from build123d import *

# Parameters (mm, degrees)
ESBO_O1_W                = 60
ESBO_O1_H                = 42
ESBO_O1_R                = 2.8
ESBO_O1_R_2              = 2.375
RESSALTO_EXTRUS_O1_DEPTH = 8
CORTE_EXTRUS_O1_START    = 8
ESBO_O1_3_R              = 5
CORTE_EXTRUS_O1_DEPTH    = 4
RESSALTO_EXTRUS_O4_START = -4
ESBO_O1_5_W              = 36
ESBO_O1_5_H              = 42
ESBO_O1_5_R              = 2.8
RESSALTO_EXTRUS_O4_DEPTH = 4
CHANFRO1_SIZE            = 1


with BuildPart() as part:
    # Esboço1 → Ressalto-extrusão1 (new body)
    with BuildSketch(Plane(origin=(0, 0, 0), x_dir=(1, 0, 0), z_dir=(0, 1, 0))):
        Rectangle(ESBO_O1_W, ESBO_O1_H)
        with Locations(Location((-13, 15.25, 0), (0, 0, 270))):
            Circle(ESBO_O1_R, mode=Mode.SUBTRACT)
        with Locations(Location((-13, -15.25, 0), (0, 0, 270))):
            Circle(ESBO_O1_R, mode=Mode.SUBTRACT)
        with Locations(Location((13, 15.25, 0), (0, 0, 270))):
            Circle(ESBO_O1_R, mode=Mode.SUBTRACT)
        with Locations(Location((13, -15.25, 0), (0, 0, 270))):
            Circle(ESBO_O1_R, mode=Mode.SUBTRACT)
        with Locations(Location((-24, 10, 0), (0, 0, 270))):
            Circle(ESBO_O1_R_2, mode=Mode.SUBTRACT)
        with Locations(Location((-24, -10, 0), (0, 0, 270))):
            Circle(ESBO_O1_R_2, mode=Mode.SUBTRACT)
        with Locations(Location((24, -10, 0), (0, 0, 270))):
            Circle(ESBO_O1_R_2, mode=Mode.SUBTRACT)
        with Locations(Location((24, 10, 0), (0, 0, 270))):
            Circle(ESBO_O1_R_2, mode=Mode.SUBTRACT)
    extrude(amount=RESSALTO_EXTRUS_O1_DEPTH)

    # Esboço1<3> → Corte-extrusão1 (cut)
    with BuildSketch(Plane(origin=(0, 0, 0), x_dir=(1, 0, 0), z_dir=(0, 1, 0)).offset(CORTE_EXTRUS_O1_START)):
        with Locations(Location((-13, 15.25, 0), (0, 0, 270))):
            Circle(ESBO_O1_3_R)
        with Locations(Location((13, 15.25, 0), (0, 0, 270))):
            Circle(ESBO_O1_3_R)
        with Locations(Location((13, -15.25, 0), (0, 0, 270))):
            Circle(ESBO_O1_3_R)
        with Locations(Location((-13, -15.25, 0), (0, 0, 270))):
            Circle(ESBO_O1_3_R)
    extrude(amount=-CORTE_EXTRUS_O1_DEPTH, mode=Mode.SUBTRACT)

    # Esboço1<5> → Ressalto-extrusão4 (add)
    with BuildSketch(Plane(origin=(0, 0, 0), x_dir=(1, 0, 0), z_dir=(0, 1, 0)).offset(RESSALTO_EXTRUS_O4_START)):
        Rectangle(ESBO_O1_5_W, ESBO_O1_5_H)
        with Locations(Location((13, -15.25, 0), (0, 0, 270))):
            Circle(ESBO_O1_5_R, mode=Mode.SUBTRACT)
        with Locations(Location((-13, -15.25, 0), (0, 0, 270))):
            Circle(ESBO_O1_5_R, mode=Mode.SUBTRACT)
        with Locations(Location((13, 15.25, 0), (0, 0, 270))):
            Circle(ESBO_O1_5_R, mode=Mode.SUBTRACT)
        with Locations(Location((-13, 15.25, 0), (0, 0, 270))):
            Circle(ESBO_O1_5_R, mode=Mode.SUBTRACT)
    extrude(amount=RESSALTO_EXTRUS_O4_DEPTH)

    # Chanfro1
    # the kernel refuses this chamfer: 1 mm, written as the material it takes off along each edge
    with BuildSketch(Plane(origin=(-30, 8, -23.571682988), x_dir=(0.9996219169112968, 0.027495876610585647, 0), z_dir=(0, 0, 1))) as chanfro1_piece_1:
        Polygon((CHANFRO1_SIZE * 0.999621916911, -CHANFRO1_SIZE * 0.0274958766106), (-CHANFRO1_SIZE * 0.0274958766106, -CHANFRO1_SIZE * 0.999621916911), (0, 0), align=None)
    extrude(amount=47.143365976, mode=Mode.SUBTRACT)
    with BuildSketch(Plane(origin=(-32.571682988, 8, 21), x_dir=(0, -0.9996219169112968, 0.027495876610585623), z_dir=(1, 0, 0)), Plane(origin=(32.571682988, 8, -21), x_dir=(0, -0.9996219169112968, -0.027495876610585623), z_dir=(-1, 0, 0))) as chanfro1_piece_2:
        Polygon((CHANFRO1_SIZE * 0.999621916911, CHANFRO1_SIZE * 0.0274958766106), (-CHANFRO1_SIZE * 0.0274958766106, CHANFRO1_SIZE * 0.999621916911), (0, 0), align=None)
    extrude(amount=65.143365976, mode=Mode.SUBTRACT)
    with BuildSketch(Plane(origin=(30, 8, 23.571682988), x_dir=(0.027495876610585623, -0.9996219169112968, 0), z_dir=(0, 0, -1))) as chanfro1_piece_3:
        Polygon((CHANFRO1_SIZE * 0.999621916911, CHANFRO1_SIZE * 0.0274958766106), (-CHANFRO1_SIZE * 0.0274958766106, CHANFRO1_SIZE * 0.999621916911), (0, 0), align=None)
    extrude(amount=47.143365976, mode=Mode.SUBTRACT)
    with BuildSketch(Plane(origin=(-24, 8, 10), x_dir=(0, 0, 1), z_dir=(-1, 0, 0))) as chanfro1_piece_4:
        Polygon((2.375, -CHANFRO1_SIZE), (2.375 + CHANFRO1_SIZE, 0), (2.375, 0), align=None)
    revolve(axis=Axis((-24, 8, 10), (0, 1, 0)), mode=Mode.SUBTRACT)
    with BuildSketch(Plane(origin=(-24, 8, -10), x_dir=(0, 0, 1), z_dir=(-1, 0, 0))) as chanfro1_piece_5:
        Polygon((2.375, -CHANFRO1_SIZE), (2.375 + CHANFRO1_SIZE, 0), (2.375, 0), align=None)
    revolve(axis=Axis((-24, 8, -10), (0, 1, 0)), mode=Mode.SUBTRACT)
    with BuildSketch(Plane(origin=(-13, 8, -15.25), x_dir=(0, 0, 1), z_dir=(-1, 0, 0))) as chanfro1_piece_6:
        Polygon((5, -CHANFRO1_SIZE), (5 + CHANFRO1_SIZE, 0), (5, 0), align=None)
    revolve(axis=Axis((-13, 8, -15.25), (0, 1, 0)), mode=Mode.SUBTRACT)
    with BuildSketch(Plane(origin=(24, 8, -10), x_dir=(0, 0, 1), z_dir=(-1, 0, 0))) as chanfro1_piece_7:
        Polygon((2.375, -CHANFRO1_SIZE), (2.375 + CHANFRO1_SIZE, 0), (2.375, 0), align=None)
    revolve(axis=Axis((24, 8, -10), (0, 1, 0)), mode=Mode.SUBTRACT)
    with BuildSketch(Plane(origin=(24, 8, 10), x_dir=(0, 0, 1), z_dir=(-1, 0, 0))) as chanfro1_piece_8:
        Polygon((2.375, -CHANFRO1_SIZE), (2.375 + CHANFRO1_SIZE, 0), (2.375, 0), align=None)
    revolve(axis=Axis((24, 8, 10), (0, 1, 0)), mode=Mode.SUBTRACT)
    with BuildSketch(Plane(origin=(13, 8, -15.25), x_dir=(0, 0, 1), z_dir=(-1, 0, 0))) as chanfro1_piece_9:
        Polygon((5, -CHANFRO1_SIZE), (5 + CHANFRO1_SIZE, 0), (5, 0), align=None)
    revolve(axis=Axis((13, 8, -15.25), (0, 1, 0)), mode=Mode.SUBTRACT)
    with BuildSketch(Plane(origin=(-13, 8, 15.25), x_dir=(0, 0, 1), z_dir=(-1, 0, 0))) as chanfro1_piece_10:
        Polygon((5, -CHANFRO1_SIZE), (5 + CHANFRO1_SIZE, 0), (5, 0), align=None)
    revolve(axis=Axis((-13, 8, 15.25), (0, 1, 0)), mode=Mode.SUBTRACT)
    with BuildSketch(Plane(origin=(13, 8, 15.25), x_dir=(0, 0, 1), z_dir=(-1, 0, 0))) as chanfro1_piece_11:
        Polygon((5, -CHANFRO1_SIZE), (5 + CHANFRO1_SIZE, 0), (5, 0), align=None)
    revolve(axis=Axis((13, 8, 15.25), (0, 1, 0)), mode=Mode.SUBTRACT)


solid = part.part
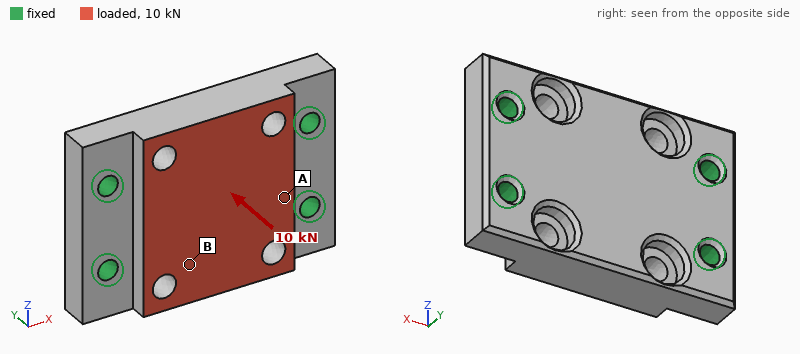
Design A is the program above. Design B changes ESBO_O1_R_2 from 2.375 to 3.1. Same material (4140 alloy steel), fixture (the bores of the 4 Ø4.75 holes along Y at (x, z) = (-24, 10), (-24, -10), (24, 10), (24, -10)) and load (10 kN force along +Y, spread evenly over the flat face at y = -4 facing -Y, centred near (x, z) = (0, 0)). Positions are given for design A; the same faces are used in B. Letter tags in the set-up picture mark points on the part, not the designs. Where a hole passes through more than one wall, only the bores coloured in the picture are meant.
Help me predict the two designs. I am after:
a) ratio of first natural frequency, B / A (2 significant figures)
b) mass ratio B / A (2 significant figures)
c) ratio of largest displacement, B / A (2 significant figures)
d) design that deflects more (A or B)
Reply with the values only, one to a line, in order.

1.1
0.98
0.85
A
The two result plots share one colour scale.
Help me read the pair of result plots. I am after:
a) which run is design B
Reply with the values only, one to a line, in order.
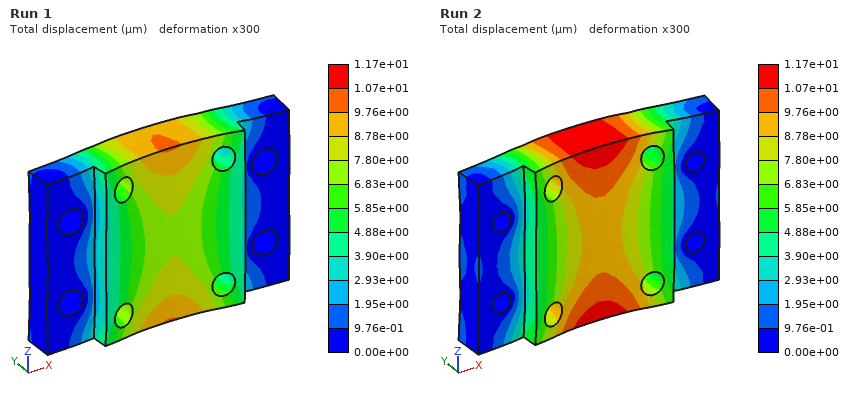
Run 1
